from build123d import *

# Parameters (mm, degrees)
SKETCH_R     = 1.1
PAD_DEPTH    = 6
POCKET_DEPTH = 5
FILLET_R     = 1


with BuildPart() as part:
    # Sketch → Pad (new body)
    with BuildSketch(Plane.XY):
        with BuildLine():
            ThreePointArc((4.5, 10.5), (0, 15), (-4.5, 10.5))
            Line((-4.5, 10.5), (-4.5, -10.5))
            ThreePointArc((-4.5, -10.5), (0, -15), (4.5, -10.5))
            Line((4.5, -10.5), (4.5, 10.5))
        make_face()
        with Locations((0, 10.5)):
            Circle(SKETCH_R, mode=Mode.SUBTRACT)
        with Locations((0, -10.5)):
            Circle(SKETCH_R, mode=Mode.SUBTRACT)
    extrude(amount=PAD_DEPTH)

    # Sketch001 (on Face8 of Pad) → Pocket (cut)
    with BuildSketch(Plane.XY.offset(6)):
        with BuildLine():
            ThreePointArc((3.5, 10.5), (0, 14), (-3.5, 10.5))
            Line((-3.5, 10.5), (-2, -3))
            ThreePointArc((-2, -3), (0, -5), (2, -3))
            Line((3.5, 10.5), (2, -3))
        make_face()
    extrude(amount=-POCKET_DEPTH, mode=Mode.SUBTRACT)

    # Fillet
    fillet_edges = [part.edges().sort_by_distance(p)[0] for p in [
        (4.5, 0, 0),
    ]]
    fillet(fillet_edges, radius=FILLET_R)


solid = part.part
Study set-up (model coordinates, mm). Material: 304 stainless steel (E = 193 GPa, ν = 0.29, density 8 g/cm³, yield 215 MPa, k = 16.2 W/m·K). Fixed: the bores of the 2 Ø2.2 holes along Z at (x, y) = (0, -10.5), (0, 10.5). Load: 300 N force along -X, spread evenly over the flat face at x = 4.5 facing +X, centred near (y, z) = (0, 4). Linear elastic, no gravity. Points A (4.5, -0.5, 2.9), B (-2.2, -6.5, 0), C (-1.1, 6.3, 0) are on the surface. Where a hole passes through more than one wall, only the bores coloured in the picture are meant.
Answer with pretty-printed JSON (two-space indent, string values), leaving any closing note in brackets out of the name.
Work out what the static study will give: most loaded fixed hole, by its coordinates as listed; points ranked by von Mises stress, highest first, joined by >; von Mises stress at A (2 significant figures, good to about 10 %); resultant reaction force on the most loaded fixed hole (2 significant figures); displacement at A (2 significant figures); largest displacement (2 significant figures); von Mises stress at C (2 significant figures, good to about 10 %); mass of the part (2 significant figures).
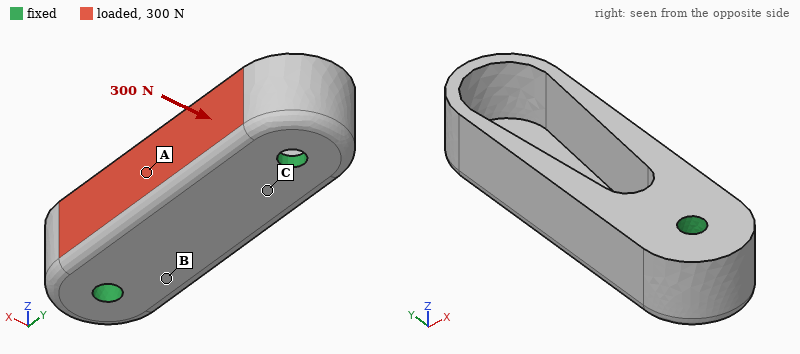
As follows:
{
  "most loaded fixed hole, by its coordinates as listed": "(0, -10.5)",
  "points ranked by von Mises stress, highest first, joined by >": "A > C > B",
  "von Mises stress at A": "46 MPa",
  "resultant reaction force on the most loaded fixed hole": "180 N",
  "displacement at A": "2.9 µm",
  "largest displacement": "9.9 µm",
  "von Mises stress at C": "21 MPa",
  "mass of the part": "7.8 g"
}
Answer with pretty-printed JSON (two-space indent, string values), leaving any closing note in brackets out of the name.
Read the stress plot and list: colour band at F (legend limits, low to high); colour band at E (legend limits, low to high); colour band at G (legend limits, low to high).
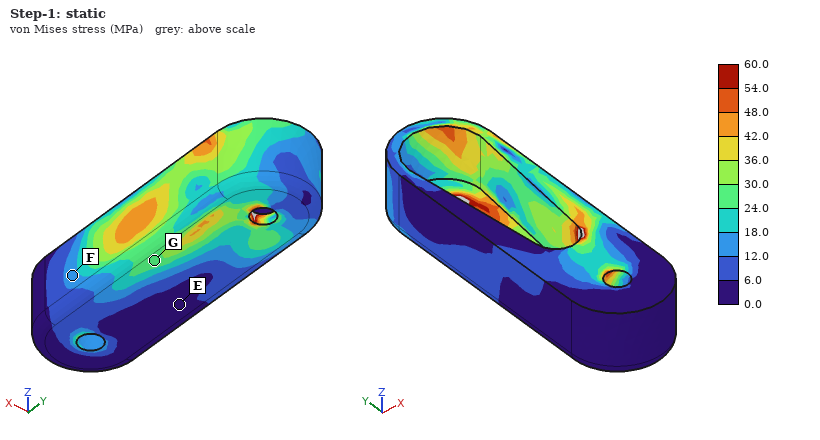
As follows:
{
  "colour band at F": "12.0 to 18.0 MPa",
  "colour band at E": "0.0 to 6.0 MPa",
  "colour band at G": "24.0 to 30.0 MPa"
}
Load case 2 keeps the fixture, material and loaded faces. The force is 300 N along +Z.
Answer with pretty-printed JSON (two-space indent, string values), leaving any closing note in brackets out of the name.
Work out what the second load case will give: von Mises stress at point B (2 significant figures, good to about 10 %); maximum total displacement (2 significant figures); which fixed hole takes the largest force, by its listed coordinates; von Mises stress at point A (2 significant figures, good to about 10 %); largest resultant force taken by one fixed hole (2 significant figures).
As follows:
{
  "von Mises stress at point B": "15 MPa",
  "maximum total displacement": "9.6 µm",
  "which fixed hole takes the largest force, by its listed coordinates": "(0, -10.5)",
  "von Mises stress at point A": "39 MPa",
  "largest resultant force taken by one fixed hole": "210 N"
}
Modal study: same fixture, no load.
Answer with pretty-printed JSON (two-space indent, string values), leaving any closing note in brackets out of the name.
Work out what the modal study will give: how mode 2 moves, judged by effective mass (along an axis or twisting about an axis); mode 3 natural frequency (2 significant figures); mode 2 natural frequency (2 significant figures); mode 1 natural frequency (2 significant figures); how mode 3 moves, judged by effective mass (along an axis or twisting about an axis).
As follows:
{
  "how mode 2 moves, judged by effective mass": "along Z",
  "mode 3 natural frequency": "34 kHz",
  "mode 2 natural frequency": "28 kHz",
  "mode 1 natural frequency": "22 kHz",
  "how mode 3 moves, judged by effective mass": "along X"
}
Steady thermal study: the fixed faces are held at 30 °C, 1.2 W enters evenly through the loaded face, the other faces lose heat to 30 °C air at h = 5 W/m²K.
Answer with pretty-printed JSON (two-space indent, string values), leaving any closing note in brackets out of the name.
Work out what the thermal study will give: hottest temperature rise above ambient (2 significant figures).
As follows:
{
  "hottest temperature rise above ambient": "15 K"
}
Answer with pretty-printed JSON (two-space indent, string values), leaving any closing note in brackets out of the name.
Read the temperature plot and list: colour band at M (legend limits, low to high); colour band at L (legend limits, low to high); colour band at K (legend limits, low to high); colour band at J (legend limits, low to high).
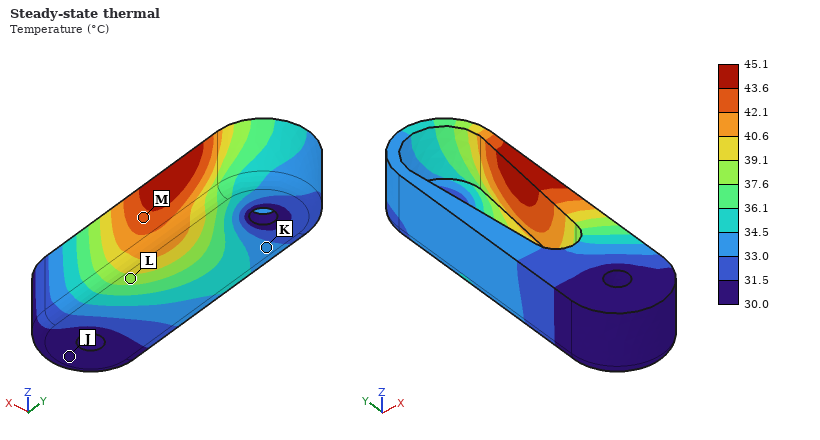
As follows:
{
  "colour band at M": "42.1 to 43.6 °C",
  "colour band at L": "37.6 to 39.1 °C",
  "colour band at K": "33.0 to 34.5 °C",
  "colour band at J": "30.0 to 31.5 °C"
}
